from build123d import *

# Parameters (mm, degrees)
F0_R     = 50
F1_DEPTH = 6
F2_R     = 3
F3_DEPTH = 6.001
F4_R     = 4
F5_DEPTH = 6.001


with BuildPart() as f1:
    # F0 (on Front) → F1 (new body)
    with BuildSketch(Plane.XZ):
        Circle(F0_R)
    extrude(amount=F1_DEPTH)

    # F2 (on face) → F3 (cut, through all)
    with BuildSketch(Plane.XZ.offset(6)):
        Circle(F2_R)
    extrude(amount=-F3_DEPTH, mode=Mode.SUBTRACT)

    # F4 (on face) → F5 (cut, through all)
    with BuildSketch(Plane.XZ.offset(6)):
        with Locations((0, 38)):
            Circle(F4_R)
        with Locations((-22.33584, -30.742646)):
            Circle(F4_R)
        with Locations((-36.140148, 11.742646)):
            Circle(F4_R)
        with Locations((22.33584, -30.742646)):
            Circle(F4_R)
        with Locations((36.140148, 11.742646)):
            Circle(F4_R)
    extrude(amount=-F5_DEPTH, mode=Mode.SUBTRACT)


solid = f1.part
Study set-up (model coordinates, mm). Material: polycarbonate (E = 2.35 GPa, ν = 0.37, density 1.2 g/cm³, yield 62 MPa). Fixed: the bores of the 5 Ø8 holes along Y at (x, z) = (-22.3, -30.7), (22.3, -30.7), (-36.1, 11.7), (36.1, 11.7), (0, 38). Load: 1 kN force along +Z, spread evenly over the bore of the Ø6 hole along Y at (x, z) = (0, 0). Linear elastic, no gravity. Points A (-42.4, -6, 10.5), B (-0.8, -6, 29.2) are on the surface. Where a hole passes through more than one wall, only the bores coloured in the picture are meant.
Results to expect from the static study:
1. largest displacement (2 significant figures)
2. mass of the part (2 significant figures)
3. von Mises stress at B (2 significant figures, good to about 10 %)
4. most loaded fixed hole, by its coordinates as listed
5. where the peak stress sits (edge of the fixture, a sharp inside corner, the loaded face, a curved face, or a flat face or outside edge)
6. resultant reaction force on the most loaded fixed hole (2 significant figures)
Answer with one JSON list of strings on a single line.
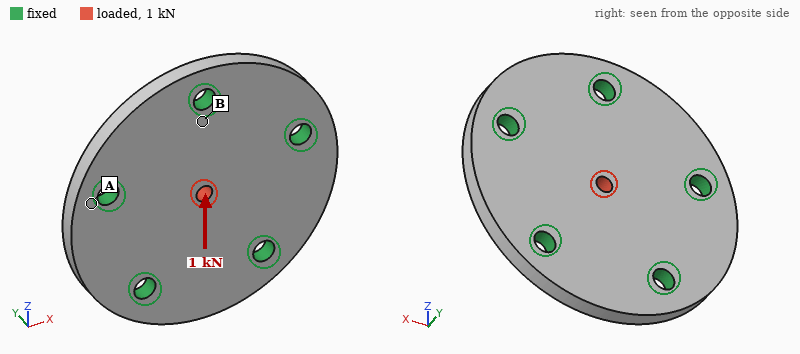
["55 µm", "55 g", "3.4 MPa", "(0, 38)", "the loaded face", "300 N"]
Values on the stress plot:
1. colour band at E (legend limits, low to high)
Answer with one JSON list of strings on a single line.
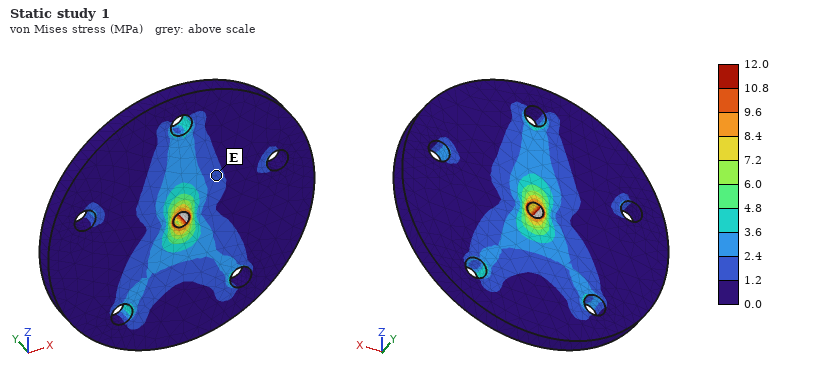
["1.2 to 2.4 MPa"]
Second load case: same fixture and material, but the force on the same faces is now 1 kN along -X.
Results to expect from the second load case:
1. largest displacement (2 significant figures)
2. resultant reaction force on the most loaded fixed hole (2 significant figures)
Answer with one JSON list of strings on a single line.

["55 µm", "290 N"]
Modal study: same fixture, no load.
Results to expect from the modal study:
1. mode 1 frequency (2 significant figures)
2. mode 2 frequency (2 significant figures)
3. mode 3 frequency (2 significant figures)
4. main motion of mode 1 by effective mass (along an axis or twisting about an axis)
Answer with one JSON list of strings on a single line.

["2500 Hz", "3200 Hz", "3200 Hz", "along Y"]
